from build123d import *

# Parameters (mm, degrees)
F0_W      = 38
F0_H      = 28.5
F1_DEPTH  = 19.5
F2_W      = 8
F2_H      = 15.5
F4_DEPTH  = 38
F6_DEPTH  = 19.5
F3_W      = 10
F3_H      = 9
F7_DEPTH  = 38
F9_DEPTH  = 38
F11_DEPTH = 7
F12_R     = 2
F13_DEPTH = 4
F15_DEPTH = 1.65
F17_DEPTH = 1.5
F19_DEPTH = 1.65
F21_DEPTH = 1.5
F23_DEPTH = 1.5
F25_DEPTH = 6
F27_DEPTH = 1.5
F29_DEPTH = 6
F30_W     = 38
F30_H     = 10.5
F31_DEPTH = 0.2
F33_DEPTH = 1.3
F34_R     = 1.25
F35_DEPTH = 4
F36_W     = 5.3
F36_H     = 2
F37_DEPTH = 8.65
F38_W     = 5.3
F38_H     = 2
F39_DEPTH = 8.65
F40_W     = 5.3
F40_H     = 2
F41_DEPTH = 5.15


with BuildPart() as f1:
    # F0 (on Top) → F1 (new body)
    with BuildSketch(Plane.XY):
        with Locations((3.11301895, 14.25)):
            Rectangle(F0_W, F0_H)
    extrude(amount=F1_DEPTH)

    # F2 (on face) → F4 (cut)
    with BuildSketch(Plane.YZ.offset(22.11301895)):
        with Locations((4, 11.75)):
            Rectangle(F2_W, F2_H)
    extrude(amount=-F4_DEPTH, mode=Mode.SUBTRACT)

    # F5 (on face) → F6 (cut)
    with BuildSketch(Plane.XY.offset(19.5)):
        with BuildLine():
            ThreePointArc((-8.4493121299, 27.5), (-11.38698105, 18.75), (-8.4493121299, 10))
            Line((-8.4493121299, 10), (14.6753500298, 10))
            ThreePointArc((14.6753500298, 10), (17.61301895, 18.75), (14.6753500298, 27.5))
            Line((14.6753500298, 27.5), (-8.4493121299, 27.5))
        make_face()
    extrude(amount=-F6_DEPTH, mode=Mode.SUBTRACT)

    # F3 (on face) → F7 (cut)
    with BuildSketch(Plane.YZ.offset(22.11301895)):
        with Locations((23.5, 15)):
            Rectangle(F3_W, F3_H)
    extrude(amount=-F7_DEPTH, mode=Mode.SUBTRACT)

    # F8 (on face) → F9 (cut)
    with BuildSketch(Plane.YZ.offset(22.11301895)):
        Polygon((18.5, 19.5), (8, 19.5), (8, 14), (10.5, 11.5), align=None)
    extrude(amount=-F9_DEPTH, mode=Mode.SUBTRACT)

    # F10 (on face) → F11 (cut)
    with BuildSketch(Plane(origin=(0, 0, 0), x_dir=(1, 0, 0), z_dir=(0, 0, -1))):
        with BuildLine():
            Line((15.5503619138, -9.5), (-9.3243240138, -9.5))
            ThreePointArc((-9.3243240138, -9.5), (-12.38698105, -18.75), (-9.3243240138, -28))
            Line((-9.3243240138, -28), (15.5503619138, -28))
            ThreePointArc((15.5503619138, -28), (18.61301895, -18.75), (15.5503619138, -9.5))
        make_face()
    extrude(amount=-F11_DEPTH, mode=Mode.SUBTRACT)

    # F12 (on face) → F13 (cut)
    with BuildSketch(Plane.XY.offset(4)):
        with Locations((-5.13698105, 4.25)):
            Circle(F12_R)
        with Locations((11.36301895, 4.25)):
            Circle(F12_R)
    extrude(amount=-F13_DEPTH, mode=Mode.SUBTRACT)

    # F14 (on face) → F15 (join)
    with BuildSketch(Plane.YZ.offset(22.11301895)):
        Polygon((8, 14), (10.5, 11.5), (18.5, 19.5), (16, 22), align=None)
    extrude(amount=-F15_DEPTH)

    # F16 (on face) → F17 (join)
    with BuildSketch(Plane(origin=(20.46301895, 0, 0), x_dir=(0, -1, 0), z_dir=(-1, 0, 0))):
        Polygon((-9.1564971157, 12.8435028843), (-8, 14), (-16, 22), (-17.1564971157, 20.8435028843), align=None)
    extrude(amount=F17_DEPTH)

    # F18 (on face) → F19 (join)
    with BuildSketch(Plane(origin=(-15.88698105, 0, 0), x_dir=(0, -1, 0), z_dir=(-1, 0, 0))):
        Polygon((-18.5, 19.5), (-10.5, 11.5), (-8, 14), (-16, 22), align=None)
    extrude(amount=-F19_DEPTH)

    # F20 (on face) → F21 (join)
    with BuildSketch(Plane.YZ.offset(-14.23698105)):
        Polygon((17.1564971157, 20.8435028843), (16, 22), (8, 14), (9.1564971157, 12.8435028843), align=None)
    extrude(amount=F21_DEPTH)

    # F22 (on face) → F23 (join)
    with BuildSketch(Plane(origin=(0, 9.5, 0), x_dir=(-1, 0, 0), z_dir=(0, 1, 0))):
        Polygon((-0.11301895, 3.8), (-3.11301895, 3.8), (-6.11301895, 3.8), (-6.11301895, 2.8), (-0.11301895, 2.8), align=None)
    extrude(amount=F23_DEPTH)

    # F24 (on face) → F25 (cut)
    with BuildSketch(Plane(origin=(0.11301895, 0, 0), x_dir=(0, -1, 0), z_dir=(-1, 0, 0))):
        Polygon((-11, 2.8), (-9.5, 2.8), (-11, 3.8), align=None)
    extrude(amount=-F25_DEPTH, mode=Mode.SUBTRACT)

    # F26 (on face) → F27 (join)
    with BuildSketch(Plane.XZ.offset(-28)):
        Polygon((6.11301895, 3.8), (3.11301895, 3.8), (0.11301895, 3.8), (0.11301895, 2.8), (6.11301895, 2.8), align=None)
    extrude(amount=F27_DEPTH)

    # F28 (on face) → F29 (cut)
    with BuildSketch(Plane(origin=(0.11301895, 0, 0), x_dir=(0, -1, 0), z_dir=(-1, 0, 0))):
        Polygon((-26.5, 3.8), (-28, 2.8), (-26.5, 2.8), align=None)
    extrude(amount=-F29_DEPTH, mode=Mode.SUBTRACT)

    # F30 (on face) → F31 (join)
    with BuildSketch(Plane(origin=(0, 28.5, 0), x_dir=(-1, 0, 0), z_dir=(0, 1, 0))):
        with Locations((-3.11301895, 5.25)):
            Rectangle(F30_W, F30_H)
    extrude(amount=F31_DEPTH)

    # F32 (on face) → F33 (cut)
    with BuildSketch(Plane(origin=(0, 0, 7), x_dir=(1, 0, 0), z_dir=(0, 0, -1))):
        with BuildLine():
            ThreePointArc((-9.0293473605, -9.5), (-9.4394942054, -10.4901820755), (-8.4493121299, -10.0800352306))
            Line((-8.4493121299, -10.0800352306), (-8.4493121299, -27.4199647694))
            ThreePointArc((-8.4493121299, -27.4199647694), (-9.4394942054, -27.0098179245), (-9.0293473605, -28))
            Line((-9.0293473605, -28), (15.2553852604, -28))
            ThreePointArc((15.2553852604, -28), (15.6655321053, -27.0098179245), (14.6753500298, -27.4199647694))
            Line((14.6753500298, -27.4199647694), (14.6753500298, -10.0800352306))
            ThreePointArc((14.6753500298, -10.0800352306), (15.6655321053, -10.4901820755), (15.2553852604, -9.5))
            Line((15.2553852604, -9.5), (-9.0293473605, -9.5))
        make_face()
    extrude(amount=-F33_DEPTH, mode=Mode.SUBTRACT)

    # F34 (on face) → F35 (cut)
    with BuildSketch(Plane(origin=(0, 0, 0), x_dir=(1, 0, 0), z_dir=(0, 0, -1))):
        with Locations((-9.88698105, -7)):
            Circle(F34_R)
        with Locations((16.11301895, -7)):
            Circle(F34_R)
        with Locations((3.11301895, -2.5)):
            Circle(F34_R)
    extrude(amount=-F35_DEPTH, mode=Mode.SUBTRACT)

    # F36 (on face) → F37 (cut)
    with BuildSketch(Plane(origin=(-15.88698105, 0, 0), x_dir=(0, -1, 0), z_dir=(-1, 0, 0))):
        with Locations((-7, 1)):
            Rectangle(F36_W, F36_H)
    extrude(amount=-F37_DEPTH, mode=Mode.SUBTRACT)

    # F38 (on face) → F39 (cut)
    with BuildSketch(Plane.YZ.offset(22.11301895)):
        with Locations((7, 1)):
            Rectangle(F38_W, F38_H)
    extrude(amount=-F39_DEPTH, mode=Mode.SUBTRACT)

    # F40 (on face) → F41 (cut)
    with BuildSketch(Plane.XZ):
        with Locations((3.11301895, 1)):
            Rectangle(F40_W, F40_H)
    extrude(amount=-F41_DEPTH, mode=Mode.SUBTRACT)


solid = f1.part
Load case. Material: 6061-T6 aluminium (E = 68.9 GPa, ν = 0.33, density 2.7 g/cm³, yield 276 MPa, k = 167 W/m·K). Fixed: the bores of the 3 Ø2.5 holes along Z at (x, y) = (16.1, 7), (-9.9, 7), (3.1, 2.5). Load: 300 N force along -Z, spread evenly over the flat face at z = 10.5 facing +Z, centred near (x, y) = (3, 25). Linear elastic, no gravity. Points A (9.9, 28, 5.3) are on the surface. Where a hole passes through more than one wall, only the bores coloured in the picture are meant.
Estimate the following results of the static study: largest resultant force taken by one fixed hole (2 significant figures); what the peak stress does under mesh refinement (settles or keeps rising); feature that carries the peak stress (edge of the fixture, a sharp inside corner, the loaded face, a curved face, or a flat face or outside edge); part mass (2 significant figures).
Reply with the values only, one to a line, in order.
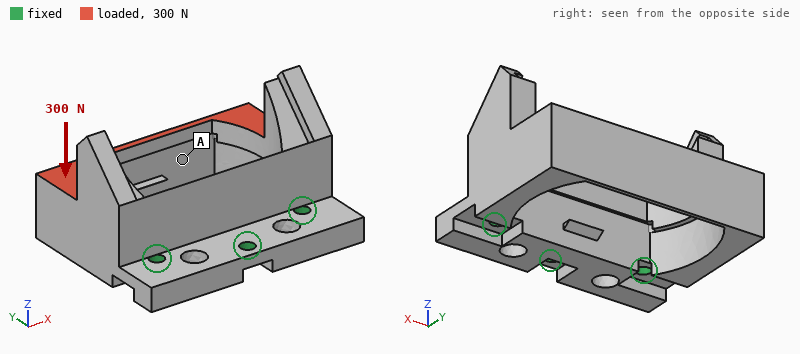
210 N
keeps rising
edge of the fixture
12 g
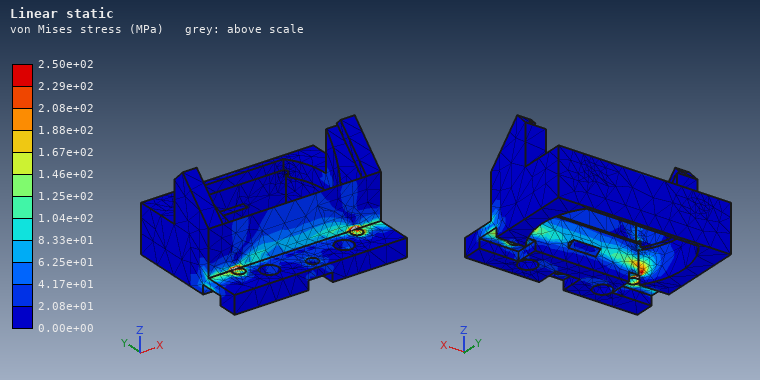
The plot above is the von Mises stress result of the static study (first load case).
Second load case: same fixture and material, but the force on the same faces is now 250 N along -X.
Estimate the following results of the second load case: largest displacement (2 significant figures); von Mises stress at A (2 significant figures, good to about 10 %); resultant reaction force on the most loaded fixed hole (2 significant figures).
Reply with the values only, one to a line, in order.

81 µm
17 MPa
200 N
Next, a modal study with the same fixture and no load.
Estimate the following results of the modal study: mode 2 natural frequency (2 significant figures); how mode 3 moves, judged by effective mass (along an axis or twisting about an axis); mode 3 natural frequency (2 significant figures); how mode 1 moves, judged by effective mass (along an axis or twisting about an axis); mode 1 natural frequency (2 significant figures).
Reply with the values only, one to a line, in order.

4600 Hz
along X
5400 Hz
along Z
2800 Hz
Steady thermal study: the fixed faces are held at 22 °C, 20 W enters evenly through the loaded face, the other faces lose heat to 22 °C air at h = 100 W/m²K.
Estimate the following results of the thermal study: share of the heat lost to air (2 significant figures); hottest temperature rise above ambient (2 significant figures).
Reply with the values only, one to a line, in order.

23 %
32 K
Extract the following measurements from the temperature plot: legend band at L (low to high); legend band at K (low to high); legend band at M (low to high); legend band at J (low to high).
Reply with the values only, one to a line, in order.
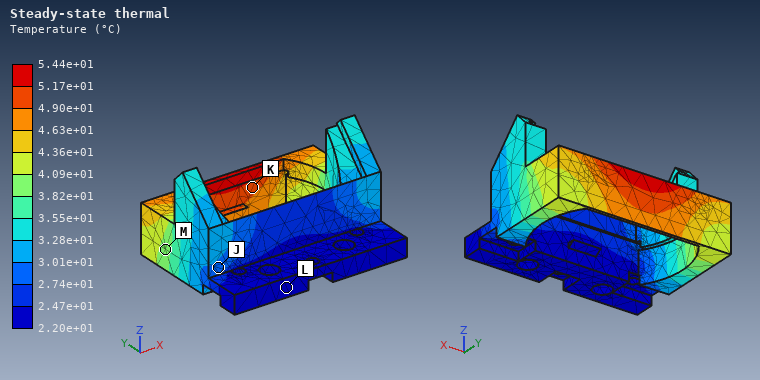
2.20e+01 to 2.47e+01 °C
4.90e+01 to 5.17e+01 °C
3.82e+01 to 4.09e+01 °C
2.74e+01 to 3.01e+01 °C
